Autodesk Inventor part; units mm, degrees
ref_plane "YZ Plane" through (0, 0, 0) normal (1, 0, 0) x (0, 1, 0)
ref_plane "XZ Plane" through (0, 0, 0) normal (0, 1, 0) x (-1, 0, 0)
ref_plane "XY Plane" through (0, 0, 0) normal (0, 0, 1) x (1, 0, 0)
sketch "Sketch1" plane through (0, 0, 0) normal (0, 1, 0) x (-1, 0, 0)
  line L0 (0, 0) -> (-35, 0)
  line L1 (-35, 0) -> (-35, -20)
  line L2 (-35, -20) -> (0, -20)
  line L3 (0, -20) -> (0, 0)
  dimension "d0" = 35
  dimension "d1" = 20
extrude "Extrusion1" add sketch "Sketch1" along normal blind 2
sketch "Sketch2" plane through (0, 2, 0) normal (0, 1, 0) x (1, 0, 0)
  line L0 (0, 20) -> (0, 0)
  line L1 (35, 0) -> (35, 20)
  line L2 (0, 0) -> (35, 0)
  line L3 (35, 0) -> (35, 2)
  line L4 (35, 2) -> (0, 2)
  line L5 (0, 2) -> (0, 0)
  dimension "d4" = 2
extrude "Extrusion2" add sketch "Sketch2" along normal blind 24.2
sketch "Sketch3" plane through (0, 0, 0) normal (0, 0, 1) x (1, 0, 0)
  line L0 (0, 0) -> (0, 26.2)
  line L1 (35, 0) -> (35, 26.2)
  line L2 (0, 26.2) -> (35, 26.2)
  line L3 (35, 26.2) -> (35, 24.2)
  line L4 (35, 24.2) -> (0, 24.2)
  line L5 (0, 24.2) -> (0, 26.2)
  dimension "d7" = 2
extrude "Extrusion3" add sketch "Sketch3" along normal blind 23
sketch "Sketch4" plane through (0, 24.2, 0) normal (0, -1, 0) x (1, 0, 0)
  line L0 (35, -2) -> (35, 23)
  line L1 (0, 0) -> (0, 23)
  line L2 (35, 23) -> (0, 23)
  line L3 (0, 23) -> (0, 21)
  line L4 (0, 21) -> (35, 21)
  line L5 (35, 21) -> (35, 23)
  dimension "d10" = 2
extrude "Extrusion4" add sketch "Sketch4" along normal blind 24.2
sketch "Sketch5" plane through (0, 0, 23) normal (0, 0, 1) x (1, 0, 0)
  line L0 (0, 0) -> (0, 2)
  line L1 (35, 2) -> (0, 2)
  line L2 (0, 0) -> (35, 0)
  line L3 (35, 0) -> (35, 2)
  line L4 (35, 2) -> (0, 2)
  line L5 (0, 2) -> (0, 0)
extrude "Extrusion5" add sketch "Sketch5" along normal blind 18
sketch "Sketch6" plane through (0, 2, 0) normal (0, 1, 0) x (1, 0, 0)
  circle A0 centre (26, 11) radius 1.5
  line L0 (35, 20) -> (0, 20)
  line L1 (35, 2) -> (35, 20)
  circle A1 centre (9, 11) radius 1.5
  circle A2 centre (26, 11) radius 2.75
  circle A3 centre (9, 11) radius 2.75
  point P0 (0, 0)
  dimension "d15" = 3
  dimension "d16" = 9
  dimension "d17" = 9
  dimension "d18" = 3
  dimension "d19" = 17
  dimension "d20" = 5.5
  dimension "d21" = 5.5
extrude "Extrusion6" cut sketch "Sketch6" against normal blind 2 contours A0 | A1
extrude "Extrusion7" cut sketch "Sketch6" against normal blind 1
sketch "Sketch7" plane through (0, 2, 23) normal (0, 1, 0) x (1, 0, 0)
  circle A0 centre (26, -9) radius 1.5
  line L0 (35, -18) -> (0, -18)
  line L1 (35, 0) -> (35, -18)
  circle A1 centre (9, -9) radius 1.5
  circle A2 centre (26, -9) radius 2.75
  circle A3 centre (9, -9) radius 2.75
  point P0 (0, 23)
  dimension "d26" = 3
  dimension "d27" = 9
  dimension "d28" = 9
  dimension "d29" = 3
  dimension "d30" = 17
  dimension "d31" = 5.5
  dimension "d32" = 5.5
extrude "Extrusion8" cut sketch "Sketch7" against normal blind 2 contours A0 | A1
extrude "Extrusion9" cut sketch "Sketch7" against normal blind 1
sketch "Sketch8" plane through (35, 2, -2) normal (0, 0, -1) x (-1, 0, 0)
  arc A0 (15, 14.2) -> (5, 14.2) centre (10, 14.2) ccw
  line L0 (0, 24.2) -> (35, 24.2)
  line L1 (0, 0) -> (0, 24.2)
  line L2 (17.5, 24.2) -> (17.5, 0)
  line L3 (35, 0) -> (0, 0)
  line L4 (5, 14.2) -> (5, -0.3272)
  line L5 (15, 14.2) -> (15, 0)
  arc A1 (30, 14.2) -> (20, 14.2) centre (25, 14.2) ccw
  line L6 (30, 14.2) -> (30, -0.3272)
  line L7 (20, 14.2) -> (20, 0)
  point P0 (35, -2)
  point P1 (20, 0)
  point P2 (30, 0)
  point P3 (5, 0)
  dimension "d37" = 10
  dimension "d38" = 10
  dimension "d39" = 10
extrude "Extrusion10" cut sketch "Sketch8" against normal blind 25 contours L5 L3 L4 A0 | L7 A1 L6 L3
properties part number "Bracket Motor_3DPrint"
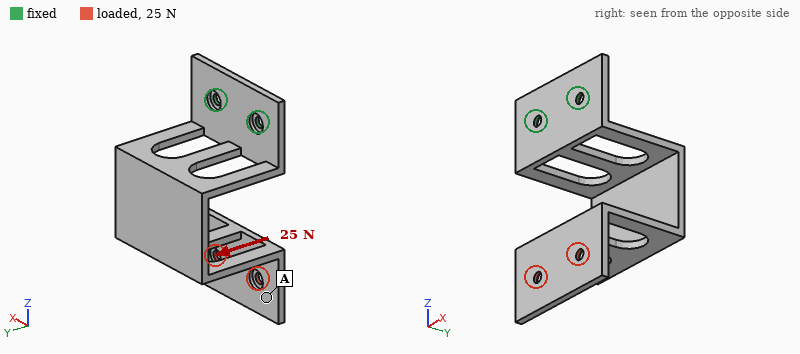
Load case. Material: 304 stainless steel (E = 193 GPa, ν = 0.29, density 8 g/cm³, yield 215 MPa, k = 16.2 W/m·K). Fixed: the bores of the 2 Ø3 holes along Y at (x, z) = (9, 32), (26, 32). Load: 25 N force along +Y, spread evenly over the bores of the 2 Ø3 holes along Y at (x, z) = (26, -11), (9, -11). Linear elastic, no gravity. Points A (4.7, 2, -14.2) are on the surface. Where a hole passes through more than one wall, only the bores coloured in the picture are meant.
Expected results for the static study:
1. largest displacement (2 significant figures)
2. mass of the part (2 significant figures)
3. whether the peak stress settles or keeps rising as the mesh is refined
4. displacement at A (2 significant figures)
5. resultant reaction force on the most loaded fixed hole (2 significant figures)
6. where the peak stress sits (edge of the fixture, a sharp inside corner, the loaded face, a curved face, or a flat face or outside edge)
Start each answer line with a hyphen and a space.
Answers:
- 0.70 mm
- 49 g
- keeps rising
- 0.59 mm
- 25 N
- edge of the fixture
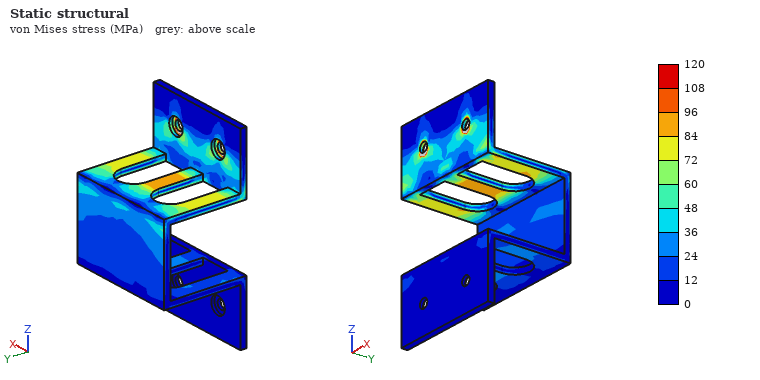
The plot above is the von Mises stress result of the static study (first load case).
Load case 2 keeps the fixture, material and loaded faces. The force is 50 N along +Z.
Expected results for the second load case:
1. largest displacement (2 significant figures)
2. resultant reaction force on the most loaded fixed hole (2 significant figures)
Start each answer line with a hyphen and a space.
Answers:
- 0.65 mm
- 26 N
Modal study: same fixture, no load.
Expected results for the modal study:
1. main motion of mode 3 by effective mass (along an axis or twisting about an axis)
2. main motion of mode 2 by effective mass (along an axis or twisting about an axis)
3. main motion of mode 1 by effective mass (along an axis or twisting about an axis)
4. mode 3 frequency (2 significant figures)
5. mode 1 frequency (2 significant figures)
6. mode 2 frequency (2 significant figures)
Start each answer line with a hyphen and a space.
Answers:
- along Z
- along X
- along Y
- 600 Hz
- 250 Hz
- 470 Hz
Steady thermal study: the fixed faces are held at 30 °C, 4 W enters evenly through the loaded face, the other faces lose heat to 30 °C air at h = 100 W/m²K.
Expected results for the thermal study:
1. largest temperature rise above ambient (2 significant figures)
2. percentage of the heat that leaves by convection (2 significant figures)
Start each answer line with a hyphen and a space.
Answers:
- 43 K
- 100 %
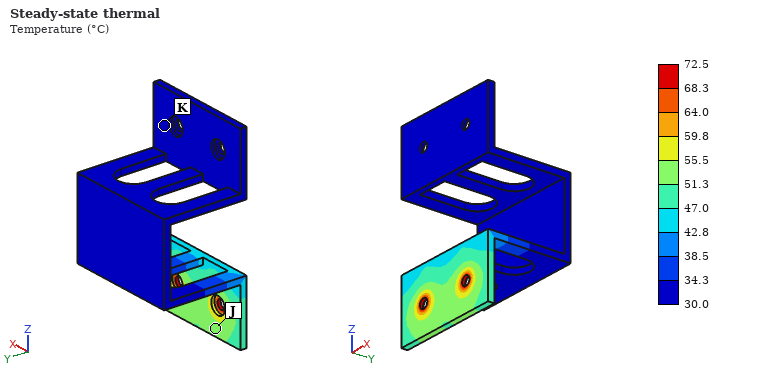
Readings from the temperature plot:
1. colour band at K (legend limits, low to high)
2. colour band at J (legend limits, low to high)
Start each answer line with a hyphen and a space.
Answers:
- 30.0 to 34.3 °C
- 51.3 to 55.5 °C
